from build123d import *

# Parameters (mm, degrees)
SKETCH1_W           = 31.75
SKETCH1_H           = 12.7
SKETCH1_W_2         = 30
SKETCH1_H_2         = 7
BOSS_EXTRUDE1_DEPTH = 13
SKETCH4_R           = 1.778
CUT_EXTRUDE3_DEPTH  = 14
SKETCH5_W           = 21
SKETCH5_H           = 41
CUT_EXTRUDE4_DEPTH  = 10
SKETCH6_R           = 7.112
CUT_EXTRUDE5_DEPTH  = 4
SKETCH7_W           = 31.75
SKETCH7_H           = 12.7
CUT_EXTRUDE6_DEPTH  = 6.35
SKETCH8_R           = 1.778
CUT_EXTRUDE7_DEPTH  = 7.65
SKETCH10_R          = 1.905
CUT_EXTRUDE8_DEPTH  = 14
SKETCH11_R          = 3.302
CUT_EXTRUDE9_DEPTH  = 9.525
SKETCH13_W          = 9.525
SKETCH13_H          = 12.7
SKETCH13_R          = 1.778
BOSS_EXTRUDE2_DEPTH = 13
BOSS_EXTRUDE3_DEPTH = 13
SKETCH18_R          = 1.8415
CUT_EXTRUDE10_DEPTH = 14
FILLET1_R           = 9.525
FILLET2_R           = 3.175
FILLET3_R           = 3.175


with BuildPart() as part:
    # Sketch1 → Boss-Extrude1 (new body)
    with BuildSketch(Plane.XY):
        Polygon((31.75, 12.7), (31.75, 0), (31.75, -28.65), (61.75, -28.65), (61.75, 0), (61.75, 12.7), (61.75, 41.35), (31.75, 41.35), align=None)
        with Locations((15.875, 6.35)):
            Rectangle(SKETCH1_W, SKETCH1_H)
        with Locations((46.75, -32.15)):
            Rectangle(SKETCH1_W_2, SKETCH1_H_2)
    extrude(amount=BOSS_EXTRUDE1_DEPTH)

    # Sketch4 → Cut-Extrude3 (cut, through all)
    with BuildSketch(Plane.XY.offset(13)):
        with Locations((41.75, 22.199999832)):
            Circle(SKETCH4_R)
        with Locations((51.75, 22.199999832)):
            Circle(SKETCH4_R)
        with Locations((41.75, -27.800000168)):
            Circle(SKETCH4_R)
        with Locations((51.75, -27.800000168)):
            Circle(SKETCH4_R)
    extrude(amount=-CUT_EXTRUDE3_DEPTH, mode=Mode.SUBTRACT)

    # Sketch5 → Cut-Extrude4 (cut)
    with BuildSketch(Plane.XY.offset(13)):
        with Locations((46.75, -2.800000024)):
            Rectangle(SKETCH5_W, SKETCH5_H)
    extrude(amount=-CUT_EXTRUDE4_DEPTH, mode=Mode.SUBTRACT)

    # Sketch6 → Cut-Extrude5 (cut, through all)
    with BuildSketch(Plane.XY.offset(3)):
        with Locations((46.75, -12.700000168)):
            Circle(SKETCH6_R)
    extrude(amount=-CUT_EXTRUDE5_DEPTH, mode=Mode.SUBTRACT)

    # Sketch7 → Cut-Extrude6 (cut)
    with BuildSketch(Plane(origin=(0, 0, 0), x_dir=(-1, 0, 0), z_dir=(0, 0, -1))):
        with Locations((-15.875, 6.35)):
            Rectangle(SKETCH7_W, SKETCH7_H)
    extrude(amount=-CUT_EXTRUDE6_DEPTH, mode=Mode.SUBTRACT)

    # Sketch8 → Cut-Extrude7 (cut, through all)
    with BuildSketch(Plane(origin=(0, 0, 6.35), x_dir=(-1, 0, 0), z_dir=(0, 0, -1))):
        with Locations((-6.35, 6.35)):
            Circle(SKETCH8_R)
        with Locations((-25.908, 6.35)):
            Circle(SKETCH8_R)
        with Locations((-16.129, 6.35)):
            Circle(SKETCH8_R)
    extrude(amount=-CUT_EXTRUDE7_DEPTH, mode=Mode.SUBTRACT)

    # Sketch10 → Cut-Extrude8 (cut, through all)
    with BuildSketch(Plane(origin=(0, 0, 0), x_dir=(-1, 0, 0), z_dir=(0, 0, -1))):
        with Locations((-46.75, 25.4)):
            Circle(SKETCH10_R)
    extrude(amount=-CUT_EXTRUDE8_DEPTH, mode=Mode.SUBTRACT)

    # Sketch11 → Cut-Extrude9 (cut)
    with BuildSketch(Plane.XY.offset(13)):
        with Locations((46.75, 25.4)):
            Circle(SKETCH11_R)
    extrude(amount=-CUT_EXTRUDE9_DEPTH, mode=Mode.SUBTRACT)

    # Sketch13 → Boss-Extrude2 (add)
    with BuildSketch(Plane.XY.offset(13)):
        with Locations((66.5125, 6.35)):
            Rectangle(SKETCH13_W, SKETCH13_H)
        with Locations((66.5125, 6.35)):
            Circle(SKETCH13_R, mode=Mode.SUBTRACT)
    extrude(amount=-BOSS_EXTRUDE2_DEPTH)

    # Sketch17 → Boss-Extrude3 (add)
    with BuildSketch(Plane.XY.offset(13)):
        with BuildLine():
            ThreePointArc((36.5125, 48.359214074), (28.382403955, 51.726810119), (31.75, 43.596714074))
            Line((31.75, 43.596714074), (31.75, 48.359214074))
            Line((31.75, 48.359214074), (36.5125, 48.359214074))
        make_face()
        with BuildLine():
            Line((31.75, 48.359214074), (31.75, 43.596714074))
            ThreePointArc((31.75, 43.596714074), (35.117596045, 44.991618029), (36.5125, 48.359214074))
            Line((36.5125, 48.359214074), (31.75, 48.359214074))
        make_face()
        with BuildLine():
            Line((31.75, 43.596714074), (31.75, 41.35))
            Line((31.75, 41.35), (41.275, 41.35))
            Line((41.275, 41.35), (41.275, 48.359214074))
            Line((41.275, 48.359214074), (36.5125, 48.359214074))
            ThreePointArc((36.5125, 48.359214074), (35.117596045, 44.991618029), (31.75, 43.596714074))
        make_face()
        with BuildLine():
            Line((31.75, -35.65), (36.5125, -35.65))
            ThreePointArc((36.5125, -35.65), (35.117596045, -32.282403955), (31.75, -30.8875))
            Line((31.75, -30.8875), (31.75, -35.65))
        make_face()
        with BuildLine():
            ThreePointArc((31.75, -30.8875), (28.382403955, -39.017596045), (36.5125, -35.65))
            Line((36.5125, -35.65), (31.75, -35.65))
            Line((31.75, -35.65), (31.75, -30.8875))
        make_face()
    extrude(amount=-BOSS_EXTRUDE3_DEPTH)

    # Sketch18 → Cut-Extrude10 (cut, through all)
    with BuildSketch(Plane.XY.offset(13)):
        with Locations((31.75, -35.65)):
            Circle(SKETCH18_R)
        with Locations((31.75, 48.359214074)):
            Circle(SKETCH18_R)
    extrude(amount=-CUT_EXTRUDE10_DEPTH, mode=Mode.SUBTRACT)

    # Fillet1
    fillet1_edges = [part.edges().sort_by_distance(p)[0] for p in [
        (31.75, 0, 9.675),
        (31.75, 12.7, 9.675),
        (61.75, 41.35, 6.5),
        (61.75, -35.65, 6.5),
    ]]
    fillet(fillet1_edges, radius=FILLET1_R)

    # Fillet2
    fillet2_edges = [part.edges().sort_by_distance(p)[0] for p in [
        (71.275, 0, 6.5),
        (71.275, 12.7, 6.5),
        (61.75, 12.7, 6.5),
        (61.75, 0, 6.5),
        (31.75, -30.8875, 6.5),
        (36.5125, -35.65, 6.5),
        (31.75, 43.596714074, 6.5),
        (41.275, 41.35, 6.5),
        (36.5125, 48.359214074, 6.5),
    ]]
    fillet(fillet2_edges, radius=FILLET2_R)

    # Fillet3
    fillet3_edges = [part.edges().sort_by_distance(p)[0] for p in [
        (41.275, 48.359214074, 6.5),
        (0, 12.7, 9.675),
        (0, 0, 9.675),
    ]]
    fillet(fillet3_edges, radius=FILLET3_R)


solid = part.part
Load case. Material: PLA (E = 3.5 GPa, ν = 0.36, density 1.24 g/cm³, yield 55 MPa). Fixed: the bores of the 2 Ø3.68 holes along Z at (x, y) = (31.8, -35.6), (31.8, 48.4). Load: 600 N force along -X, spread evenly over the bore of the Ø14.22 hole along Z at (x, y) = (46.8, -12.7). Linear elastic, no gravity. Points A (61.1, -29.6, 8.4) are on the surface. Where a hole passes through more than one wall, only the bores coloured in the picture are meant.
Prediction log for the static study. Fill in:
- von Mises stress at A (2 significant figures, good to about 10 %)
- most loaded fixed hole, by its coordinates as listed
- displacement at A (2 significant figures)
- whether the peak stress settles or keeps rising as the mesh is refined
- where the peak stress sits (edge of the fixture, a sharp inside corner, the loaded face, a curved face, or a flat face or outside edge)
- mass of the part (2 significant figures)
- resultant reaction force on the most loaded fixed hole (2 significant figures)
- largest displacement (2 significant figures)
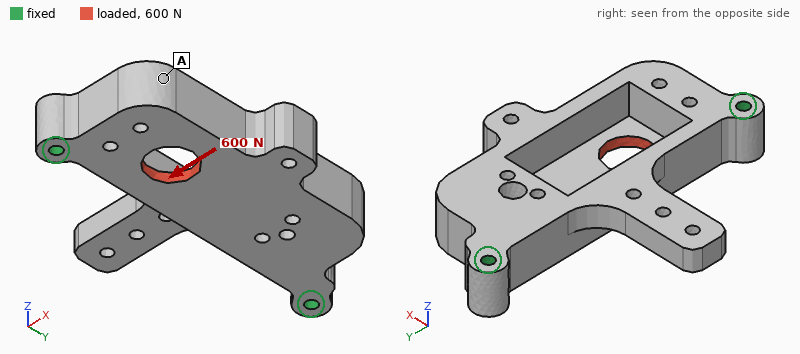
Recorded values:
2.1 MPa
(31.8, -35.6)
0.13 mm
keeps rising
edge of the fixture
32 g
490 N
0.21 mm
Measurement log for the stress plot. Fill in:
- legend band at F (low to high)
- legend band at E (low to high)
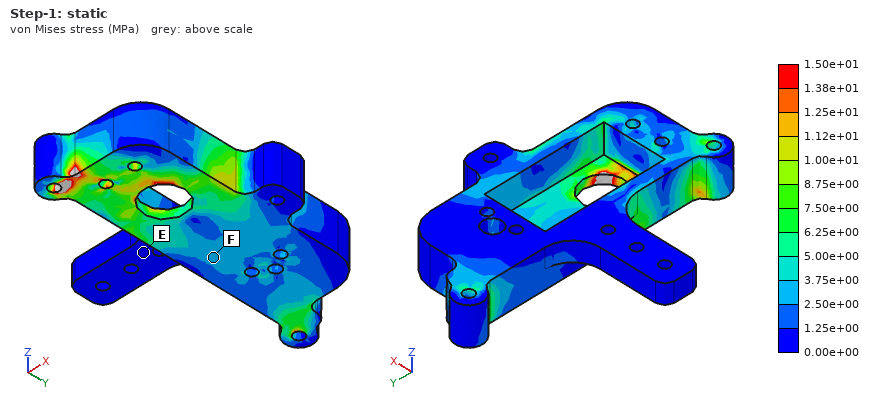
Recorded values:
2.50e+00 to 3.75e+00 MPa
0.00e+00 to 1.25e+00 MPa
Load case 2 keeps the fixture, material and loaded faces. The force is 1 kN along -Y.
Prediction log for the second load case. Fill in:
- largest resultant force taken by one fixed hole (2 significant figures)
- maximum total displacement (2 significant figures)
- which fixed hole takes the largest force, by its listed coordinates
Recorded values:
580 N
0.13 mm
(31.8, -35.6)
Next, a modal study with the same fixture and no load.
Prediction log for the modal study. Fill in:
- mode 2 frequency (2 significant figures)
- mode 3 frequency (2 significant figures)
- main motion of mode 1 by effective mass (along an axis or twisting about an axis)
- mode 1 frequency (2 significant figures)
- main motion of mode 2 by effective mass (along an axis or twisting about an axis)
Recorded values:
1300 Hz
2300 Hz
twisting about Y
990 Hz
along Z
